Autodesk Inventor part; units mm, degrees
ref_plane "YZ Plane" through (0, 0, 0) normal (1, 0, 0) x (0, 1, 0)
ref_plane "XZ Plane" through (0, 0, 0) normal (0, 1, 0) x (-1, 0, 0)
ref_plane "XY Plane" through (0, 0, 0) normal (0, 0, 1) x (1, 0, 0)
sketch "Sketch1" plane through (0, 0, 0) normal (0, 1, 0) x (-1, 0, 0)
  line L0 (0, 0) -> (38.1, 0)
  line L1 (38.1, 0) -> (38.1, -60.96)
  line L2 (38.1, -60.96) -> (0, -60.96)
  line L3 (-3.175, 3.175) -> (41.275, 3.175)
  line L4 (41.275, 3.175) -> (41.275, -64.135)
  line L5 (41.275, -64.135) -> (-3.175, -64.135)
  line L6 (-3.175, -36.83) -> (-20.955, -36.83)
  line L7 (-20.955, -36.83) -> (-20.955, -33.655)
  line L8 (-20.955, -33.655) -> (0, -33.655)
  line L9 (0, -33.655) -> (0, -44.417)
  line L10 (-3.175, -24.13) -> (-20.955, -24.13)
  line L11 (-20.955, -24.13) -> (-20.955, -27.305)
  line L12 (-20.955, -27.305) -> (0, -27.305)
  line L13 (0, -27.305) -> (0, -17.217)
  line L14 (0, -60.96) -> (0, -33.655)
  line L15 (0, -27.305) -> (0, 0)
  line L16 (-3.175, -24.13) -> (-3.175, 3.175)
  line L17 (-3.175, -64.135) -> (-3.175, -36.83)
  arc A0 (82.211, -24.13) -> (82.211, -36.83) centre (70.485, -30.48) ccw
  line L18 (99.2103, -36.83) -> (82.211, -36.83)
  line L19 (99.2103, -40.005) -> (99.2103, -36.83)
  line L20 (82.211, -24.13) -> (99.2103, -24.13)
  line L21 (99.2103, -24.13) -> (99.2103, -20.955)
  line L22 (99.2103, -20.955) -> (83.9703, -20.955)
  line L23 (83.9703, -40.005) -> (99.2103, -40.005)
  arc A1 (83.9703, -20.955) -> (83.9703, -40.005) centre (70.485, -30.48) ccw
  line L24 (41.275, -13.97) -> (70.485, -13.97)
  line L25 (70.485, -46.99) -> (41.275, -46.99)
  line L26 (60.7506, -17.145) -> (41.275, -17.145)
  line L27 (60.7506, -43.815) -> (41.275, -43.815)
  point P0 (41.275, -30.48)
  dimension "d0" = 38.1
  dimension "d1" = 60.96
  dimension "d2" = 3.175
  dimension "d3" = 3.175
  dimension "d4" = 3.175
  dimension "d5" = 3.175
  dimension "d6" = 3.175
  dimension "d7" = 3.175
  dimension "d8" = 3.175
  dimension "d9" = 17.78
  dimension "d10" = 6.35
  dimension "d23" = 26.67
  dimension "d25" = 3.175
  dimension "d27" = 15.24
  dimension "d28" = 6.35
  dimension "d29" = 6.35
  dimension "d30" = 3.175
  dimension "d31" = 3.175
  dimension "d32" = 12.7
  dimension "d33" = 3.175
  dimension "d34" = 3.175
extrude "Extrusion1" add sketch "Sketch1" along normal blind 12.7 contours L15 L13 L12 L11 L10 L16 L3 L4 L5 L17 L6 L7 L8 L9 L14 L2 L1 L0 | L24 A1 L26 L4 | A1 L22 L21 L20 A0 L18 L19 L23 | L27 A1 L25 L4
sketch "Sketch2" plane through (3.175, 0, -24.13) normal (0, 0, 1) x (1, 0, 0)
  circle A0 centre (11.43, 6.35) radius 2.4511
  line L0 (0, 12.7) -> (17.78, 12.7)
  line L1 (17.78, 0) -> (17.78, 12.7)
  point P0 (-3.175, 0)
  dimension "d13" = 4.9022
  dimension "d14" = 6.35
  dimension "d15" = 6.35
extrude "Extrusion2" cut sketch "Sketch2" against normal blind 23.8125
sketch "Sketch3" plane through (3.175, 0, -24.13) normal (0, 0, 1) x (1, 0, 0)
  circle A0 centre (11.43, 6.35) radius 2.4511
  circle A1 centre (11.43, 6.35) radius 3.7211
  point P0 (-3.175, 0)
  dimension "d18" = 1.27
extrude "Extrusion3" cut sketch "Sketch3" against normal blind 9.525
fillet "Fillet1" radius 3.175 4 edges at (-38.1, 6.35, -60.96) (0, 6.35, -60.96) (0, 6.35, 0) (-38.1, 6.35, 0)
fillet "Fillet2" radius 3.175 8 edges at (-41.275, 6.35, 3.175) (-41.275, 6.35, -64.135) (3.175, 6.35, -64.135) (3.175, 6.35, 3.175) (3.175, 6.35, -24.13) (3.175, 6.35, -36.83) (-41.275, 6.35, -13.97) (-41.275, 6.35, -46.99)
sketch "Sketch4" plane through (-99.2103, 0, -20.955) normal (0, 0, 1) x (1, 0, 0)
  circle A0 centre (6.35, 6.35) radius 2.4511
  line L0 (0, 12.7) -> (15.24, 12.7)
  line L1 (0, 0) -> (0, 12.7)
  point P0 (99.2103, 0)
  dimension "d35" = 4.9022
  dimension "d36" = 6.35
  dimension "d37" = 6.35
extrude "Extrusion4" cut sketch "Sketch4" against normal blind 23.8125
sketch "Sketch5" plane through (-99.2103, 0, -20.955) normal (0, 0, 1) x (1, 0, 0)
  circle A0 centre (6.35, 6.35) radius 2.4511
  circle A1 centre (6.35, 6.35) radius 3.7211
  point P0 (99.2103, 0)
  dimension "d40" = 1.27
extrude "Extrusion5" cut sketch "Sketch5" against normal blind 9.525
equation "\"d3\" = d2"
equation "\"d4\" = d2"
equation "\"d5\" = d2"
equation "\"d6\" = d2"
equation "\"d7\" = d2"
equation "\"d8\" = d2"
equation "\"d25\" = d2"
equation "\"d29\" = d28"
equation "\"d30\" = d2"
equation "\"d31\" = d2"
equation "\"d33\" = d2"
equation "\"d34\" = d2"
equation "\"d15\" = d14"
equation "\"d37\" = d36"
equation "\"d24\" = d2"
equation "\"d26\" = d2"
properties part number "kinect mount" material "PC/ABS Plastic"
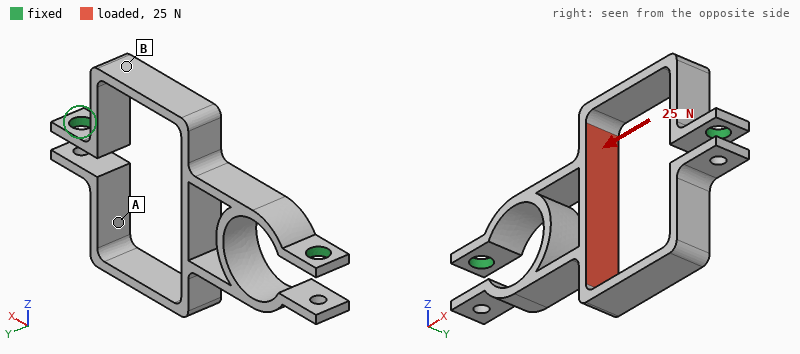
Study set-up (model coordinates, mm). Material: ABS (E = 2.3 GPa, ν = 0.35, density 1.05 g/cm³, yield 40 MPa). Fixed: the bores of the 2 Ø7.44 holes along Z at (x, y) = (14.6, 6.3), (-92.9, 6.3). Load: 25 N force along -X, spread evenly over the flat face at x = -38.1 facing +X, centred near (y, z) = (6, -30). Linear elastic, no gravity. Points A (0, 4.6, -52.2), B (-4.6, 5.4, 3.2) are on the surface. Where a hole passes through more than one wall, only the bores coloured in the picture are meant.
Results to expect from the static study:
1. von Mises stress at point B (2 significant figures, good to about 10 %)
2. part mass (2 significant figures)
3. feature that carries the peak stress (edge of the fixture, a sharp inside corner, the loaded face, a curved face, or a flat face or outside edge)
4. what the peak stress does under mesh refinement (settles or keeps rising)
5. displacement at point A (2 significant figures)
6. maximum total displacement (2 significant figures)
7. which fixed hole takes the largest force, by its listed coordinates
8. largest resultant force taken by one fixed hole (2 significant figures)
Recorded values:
1.7 MPa
16 g
edge of the fixture
keeps rising
1.4 mm
1.6 mm
(-92.9, 6.3)
29 N
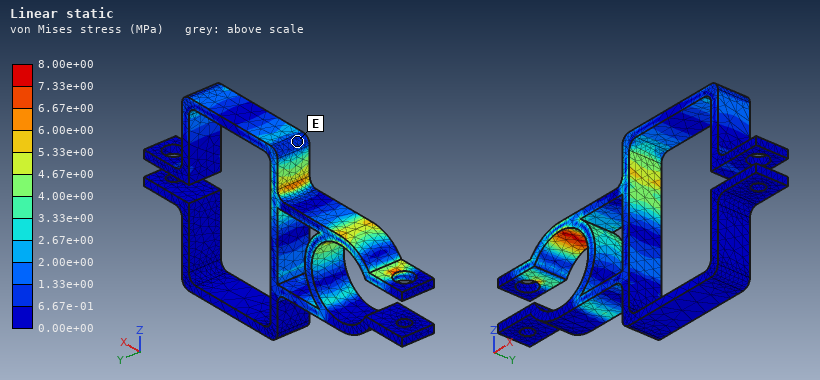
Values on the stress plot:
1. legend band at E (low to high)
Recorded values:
6.67e-01 to 1.33e+00 MPa
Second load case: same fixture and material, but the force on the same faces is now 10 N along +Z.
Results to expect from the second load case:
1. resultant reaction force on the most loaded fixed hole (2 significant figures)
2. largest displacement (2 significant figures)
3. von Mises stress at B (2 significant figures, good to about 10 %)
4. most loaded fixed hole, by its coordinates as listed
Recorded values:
7.8 N
1.5 mm
3.0 MPa
(-92.9, 6.3)
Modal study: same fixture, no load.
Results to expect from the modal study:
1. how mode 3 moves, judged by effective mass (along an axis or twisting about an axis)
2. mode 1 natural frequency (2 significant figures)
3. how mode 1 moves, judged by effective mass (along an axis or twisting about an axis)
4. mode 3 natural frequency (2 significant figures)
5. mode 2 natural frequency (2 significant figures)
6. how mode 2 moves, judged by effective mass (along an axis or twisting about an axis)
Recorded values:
along X
84 Hz
along Y
180 Hz
93 Hz
along Z
